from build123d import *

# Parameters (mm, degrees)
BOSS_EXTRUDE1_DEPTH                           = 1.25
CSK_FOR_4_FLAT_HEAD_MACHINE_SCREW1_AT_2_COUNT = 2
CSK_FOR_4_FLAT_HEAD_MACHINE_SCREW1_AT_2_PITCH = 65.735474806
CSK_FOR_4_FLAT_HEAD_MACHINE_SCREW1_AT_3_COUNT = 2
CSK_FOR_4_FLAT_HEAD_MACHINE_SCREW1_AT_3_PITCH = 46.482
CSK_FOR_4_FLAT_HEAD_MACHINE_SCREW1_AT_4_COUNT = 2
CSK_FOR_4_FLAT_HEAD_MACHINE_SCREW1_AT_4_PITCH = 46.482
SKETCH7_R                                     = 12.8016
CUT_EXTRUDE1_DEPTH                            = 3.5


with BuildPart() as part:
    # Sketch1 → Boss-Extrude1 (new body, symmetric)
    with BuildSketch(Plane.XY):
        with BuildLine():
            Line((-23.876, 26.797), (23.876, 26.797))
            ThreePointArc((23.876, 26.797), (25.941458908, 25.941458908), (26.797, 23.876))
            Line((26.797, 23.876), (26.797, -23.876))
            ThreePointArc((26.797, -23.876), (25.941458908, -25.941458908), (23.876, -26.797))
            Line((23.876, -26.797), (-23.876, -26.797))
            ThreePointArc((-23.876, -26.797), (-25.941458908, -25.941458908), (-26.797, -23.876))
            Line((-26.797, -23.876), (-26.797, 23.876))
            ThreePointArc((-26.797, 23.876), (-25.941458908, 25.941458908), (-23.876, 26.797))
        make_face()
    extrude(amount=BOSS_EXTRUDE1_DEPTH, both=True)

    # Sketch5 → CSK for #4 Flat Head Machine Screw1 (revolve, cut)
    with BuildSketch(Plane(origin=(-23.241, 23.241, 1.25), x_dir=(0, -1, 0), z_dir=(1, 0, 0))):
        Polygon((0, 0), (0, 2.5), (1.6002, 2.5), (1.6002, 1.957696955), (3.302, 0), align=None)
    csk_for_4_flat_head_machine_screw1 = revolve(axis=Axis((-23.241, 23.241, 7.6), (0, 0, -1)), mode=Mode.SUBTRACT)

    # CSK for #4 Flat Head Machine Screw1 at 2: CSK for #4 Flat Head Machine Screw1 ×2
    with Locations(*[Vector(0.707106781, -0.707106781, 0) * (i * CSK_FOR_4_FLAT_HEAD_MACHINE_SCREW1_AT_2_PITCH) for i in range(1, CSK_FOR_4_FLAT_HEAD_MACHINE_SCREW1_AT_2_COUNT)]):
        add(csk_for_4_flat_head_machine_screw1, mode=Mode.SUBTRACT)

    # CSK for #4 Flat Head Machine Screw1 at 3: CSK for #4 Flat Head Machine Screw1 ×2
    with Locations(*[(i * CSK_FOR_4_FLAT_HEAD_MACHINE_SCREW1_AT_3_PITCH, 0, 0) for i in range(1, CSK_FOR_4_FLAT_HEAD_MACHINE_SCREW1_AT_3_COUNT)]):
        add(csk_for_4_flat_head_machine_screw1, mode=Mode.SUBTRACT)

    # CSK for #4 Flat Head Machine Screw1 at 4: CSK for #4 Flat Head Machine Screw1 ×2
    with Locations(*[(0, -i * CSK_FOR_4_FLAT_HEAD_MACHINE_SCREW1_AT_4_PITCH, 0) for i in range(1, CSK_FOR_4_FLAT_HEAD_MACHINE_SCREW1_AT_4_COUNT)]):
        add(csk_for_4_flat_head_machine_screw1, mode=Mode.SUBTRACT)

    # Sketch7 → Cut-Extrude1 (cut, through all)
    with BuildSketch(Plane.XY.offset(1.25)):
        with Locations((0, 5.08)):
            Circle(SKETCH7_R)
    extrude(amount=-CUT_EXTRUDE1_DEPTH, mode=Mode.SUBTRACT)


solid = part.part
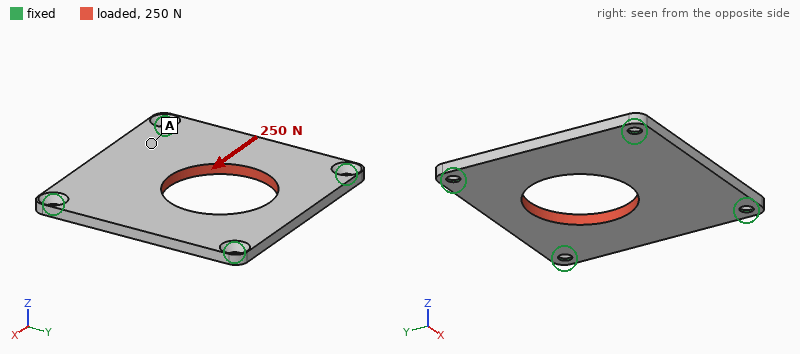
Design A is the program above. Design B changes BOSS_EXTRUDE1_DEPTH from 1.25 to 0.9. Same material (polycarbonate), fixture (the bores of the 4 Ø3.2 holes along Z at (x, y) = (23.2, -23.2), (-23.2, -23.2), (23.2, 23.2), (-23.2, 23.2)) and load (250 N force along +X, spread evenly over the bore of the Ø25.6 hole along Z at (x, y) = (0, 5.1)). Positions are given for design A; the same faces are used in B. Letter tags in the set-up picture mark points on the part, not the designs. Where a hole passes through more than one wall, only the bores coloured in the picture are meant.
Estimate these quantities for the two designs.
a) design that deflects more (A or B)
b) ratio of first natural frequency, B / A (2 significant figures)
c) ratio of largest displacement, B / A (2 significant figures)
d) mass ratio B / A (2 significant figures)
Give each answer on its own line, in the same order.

B
0.74
1.8
0.72
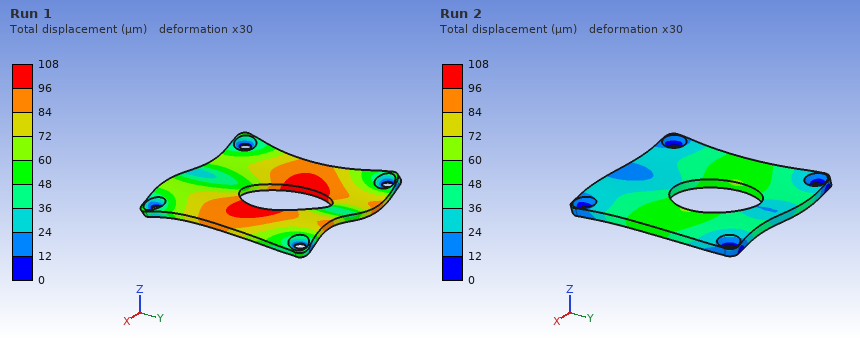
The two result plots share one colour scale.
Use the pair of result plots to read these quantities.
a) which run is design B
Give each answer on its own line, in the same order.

Run 1
